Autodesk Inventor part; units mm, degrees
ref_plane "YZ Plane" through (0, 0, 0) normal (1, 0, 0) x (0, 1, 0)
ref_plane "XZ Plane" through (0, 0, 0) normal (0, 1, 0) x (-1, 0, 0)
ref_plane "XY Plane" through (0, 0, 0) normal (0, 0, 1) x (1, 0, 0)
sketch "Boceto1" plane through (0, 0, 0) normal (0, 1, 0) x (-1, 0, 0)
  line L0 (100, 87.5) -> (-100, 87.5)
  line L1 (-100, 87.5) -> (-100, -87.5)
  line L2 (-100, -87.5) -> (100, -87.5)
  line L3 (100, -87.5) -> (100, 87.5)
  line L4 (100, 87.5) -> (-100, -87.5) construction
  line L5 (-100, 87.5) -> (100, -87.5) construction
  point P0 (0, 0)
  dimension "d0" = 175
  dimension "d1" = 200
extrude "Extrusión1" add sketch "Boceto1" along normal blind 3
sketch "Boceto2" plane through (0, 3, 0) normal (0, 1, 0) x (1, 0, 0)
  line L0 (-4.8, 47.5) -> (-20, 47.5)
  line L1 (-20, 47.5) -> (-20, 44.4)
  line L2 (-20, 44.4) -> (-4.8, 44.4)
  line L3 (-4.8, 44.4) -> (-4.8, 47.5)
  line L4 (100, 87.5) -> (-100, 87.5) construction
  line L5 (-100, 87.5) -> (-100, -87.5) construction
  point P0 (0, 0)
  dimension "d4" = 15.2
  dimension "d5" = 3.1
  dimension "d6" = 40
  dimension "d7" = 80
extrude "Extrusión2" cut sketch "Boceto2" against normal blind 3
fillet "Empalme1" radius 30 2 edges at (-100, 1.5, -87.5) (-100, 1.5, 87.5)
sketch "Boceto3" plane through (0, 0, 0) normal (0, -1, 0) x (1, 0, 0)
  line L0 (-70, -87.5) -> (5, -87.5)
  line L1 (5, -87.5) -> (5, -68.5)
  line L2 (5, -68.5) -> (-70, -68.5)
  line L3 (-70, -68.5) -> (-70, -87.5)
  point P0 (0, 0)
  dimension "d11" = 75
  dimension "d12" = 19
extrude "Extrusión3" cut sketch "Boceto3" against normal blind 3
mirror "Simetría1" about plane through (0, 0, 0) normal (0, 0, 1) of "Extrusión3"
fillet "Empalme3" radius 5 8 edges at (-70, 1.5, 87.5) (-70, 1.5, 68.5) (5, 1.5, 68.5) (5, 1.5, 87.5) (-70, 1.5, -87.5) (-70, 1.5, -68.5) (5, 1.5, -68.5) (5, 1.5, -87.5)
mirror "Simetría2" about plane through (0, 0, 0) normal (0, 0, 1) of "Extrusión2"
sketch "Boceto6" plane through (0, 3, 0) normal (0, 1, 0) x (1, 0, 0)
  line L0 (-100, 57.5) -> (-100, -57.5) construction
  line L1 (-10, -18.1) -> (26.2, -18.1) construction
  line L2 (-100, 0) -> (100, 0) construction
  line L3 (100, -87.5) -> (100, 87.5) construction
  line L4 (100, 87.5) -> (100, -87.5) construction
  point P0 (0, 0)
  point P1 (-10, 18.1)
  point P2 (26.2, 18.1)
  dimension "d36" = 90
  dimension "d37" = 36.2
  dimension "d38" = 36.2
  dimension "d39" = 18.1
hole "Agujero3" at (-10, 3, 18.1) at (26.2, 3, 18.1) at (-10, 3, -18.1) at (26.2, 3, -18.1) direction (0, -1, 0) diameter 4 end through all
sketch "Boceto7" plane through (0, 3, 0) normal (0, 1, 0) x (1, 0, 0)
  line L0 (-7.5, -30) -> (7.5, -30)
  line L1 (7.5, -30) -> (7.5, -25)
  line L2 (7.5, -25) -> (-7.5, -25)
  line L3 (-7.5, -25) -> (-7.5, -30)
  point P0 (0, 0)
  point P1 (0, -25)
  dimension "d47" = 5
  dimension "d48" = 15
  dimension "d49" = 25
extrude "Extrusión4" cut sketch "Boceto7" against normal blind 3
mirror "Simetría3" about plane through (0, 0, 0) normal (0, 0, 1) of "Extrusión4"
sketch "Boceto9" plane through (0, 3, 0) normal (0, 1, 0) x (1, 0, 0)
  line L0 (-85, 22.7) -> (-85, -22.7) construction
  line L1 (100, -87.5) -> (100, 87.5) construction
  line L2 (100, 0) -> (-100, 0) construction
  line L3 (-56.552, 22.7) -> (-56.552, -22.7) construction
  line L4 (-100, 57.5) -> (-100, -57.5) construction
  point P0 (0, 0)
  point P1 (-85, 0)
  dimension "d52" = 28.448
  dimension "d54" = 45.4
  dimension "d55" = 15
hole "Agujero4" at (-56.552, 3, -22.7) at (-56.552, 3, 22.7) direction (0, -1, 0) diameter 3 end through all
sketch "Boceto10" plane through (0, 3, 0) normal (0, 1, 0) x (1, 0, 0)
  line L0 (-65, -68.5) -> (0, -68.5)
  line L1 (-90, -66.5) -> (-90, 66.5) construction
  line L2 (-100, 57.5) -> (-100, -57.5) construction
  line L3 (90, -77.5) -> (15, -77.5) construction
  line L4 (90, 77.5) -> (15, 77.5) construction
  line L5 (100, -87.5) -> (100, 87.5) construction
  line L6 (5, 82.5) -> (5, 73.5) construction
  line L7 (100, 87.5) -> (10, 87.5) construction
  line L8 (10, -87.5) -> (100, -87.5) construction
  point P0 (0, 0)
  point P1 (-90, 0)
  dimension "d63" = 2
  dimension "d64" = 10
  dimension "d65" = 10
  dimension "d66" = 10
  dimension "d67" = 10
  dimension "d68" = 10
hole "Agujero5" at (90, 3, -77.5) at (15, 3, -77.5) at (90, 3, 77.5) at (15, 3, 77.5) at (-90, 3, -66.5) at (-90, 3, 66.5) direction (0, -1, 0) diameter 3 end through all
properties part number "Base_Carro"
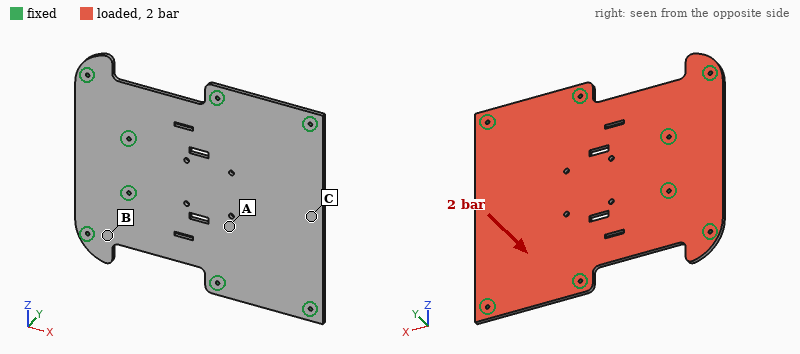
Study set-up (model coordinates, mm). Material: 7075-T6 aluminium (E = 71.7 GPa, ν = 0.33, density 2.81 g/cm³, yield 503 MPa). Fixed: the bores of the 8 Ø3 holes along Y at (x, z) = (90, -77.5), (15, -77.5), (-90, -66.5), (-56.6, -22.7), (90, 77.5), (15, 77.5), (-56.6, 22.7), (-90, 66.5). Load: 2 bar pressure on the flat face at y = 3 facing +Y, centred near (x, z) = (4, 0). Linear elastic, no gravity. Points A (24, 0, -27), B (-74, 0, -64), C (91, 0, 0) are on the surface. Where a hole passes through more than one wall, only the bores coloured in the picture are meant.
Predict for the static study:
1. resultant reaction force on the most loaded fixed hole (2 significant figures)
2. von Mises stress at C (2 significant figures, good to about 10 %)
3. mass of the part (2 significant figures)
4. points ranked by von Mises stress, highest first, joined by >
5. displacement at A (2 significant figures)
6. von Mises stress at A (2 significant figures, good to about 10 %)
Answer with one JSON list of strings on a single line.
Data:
["1.1 kN", "160 MPa", "260 g", "C > A > B", "1.6 mm", "88 MPa"]
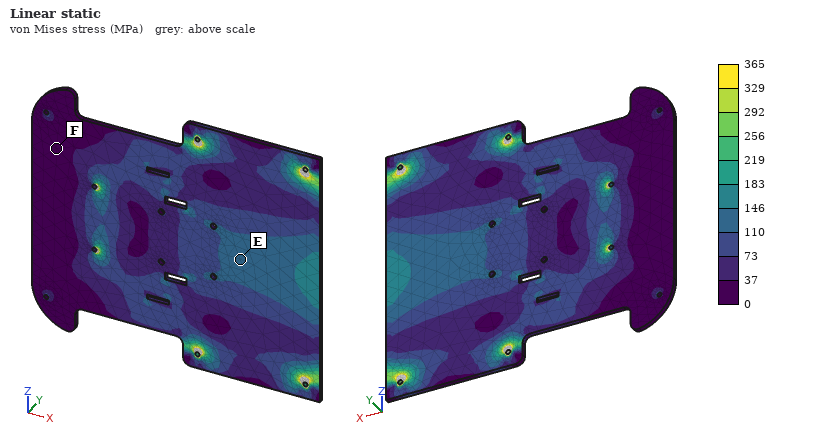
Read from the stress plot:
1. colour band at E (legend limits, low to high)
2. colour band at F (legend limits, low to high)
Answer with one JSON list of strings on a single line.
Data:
["110 to 146 MPa", "0 to 37 MPa"]
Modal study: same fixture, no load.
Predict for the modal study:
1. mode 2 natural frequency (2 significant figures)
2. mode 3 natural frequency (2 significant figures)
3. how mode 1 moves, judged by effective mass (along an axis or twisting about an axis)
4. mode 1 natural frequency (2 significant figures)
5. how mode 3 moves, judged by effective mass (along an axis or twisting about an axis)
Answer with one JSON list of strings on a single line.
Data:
["1100 Hz", "1500 Hz", "along Y", "600 Hz", "twisting about X"]
